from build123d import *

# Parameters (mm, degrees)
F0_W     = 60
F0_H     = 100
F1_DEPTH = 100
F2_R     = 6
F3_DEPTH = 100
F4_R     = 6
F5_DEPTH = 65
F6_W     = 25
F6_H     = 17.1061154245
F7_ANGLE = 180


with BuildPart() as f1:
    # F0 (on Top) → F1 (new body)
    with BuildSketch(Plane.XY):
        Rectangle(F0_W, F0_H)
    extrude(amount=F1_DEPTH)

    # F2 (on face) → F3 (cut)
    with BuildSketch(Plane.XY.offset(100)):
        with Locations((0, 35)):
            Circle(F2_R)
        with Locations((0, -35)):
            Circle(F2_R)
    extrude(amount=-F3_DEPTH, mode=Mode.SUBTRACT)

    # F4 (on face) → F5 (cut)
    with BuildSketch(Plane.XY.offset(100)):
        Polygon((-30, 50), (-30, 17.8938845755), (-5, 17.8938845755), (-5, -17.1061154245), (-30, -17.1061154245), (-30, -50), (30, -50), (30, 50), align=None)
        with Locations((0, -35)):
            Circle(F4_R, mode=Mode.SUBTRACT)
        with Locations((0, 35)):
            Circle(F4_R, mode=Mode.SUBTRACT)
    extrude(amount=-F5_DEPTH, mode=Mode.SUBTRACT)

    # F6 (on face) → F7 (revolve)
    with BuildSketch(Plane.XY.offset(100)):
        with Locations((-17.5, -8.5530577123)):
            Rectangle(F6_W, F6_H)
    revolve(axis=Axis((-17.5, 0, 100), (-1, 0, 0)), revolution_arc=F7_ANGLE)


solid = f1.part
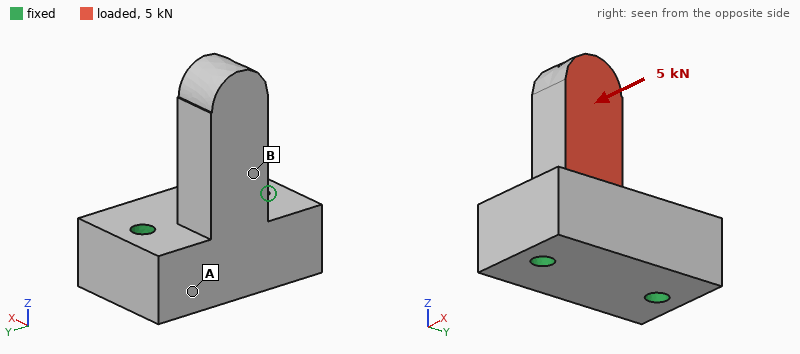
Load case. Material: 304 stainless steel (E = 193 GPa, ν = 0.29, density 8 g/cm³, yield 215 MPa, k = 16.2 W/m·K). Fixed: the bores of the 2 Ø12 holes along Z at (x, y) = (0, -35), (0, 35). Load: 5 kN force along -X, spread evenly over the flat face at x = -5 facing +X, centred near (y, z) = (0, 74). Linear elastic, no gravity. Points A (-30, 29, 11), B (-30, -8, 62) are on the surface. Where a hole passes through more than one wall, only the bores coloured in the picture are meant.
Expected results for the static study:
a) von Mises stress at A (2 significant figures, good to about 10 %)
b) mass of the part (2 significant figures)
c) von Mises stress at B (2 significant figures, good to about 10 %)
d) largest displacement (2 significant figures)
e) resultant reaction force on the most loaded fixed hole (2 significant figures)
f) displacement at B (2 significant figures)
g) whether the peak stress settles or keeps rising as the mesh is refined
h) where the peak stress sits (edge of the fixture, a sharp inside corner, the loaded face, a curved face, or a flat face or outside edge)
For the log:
10 MPa
2.2 kg
23 MPa
72 µm
2.6 kN
24 µm
keeps rising
a sharp inside corner
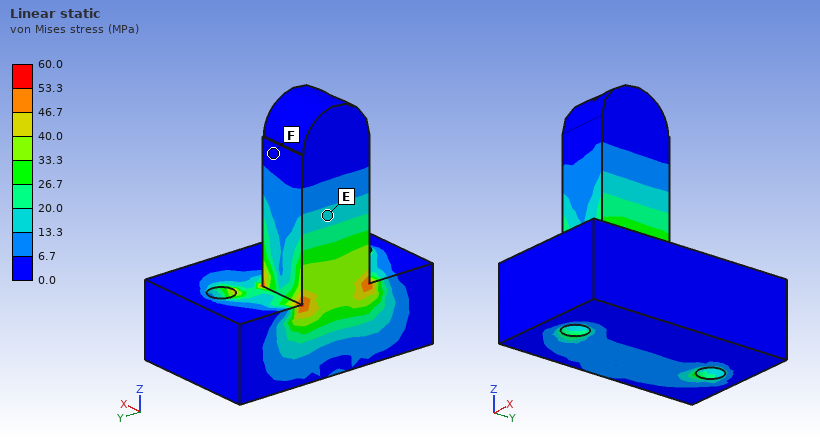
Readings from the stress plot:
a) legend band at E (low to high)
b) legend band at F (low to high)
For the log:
13.3 to 20.0 MPa
0.0 to 6.7 MPa
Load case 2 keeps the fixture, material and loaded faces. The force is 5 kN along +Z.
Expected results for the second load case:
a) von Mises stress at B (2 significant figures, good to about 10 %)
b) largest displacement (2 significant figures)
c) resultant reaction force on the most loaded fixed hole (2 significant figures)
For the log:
7.4 MPa
20 µm
2.6 kN
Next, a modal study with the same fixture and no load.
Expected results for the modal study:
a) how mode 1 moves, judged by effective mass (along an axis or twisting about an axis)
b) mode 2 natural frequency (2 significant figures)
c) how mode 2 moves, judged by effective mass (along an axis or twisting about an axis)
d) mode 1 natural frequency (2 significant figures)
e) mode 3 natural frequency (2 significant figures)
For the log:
along X
3200 Hz
along Y
2300 Hz
8300 Hz
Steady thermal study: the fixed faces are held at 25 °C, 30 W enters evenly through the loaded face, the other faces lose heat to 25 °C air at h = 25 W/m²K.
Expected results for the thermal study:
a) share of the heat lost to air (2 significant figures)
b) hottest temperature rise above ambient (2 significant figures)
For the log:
40 %
75 K
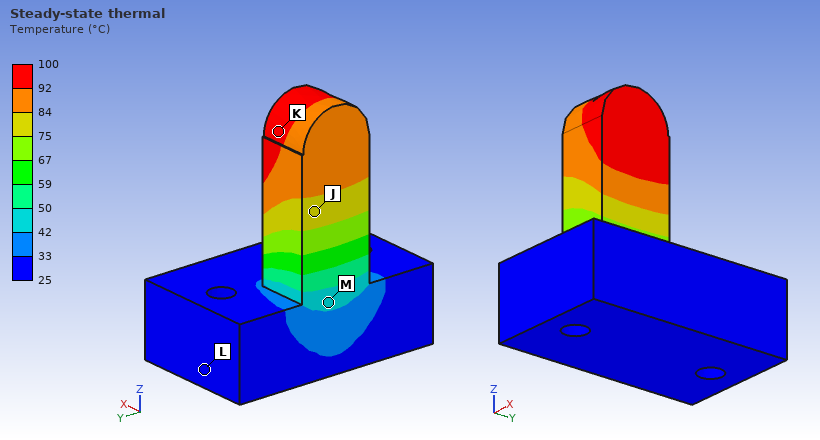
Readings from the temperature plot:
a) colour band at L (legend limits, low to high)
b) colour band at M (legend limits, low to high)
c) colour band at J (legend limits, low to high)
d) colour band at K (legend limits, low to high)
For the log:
25 to 33 °C
42 to 50 °C
75 to 84 °C
92 to 100 °C
